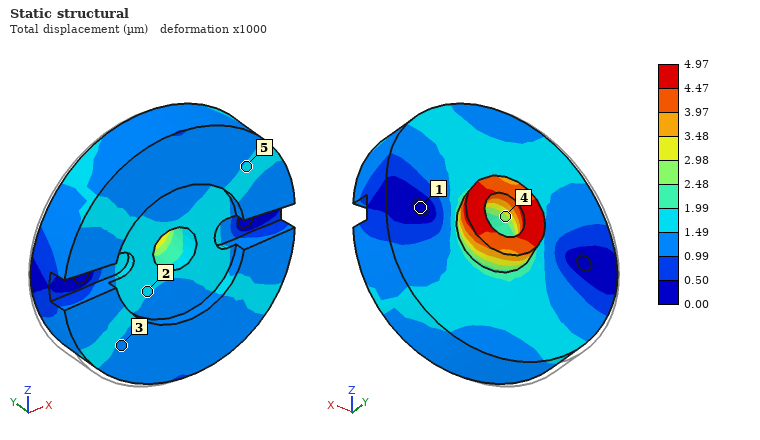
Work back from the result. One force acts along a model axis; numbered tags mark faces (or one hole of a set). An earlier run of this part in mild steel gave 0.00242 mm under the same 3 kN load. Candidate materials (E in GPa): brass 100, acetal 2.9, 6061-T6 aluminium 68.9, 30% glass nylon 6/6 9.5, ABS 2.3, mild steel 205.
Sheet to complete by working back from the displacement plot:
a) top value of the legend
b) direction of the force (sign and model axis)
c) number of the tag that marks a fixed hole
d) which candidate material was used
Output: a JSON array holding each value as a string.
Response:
["4.97 µm", "+X", "1", "brass"]
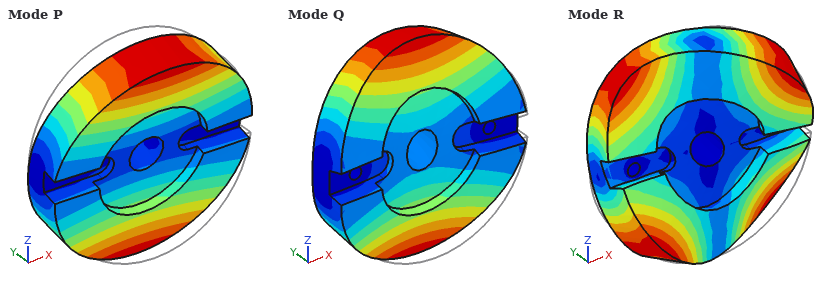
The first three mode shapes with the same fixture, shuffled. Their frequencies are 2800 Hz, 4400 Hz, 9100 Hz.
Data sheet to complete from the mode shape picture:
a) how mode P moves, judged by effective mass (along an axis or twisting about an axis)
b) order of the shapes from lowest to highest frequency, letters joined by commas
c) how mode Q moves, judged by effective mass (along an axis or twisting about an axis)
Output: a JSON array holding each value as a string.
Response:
["twisting about X", "P, Q, R", "along Y"]
